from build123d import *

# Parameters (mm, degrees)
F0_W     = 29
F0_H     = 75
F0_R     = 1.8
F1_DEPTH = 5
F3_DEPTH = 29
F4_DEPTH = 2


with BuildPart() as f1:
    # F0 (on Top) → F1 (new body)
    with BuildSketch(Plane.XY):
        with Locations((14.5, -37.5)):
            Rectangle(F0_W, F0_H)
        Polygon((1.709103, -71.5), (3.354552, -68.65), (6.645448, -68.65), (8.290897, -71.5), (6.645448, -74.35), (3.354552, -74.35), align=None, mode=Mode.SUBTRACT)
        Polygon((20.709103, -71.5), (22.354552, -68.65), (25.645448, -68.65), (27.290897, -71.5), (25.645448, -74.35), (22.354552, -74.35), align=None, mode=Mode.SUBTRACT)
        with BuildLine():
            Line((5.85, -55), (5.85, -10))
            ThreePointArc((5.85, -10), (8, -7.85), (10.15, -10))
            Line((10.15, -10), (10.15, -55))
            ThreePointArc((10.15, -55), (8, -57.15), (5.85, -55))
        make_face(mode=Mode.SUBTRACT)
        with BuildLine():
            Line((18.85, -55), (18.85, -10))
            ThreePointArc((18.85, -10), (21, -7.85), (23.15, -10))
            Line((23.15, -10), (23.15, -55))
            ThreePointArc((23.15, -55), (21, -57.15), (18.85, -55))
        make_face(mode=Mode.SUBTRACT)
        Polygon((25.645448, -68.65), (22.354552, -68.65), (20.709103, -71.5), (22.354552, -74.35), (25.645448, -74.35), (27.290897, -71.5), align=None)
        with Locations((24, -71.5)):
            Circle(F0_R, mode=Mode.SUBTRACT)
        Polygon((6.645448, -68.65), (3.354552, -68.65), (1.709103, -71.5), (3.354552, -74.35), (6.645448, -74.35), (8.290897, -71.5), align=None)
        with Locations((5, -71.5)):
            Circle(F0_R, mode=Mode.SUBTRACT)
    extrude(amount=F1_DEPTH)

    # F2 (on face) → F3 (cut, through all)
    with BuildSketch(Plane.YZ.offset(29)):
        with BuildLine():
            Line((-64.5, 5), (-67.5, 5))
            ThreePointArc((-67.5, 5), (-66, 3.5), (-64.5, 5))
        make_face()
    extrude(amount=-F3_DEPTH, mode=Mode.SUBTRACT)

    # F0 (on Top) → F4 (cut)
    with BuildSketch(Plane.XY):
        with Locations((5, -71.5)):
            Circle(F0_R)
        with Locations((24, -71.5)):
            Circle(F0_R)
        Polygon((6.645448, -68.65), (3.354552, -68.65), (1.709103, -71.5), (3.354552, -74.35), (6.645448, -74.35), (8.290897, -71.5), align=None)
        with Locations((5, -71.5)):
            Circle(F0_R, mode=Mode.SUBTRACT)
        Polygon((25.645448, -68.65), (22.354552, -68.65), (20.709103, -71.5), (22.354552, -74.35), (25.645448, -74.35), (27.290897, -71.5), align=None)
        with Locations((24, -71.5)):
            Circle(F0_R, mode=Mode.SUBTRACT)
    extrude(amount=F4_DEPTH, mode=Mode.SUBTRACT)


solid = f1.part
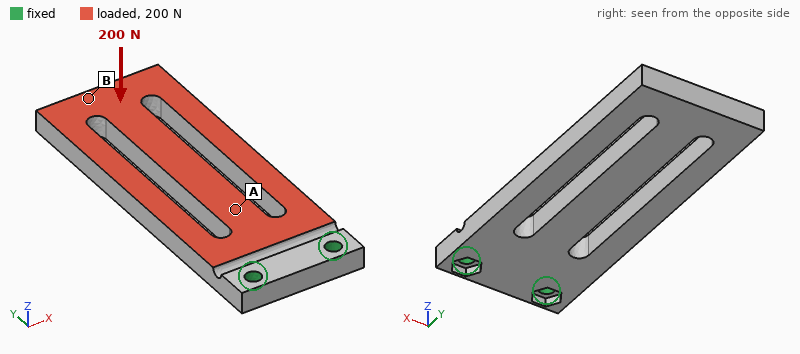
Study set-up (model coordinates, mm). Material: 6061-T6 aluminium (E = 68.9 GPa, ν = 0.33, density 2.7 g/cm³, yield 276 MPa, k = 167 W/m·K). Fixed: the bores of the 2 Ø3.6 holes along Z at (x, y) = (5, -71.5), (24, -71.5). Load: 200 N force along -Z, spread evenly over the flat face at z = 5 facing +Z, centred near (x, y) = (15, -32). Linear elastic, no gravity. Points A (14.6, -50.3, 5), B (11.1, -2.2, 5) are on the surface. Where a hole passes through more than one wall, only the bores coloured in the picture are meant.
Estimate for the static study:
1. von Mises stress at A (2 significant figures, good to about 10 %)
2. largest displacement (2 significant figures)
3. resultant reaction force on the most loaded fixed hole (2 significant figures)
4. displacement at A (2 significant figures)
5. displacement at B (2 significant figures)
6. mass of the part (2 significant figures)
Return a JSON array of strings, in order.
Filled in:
["47 MPa", "0.89 mm", "110 N", "0.16 mm", "0.85 mm", "23 g"]
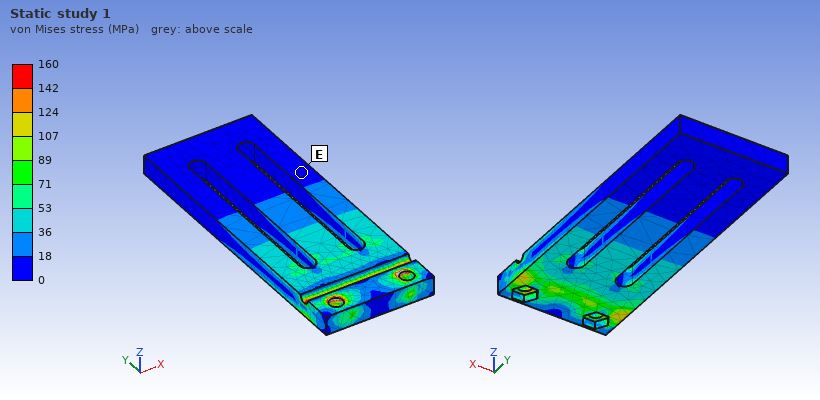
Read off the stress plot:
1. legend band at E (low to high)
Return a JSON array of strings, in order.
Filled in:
["0 to 18 MPa"]
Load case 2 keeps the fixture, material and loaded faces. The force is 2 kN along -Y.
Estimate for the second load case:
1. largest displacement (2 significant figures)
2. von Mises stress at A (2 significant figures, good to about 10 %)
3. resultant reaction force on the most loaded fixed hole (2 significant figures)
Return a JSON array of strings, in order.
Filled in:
["0.74 mm", "59 MPa", "1.0 kN"]
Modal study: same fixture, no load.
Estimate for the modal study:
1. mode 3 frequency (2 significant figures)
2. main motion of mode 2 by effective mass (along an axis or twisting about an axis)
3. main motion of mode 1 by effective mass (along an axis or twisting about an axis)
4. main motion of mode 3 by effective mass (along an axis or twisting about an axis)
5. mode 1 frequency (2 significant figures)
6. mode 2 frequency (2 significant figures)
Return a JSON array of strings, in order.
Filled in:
["2900 Hz", "along X", "along Z", "twisting about Y", "660 Hz", "2300 Hz"]
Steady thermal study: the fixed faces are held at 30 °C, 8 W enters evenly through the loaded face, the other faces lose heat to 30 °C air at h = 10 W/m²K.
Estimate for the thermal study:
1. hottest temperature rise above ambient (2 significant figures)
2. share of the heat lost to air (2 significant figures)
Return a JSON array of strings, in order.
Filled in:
["17 K", "5.2 %"]
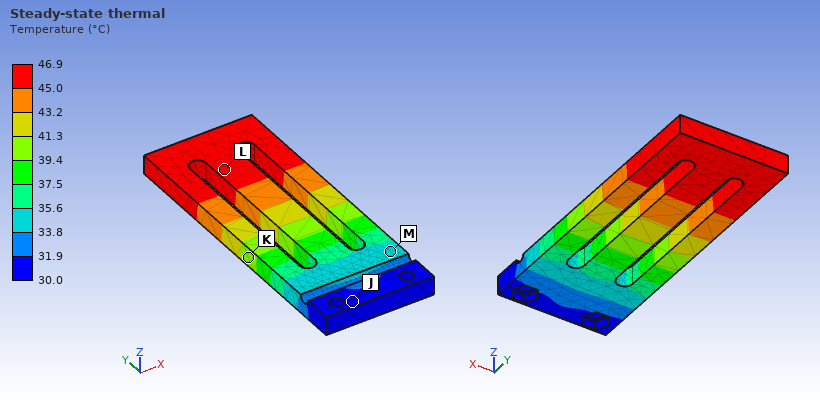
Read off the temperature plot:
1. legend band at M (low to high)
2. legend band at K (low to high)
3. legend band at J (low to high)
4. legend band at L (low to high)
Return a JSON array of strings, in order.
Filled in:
["33.8 to 35.6 °C", "39.4 to 41.3 °C", "30.0 to 31.9 °C", "45.0 to 46.9 °C"]
